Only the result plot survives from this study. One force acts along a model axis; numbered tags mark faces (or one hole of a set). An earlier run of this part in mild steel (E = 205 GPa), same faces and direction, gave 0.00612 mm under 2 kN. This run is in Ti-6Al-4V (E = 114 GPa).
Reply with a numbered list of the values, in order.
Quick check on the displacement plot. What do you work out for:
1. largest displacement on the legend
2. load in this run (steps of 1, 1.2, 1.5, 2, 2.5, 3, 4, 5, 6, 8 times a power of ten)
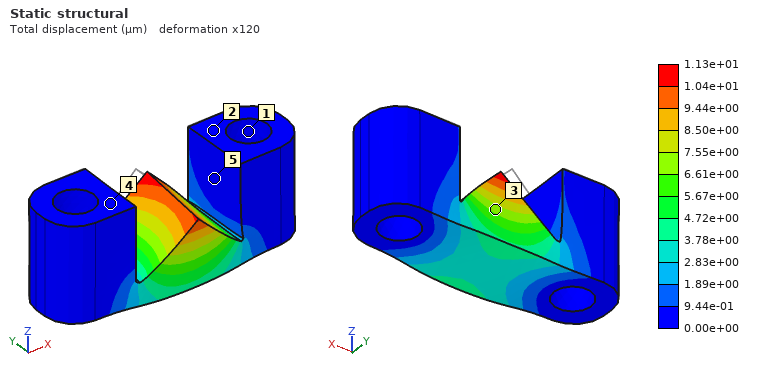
1. 1.13e+01 µm
2. 2 kN
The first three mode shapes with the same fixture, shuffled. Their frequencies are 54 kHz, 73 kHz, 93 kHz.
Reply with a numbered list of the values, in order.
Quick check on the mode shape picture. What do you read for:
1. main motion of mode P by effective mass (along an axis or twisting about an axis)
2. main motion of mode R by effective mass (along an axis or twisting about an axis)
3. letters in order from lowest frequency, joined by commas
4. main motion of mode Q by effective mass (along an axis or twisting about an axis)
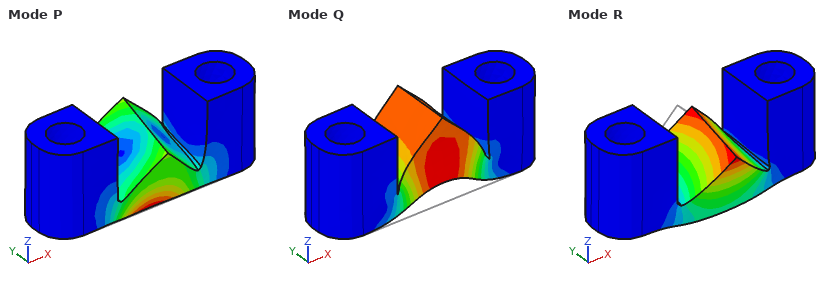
1. along Y
2. along Y
3. R, Q, P
4. along Z
